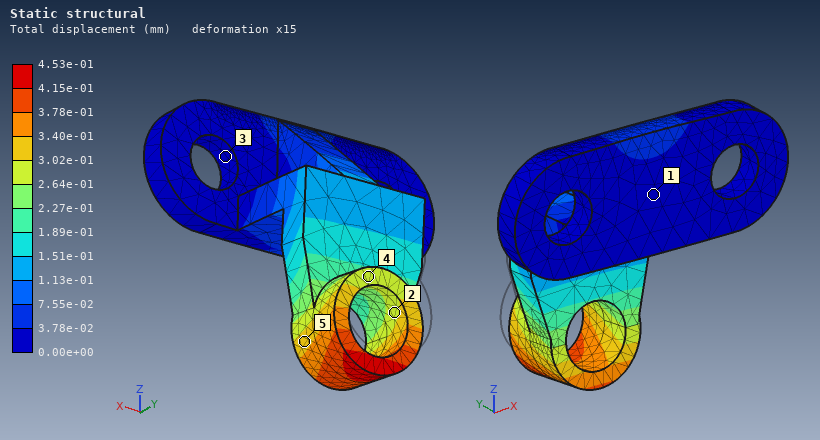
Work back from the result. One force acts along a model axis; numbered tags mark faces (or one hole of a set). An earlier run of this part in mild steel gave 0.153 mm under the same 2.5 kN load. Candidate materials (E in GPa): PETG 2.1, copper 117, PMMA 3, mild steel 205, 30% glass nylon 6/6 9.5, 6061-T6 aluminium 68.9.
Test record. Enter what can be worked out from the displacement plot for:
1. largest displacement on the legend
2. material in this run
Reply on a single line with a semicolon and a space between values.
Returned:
4.53e-01 mm; 6061-T6 aluminium
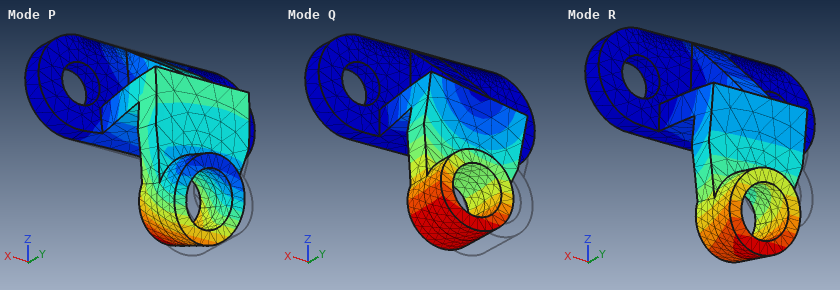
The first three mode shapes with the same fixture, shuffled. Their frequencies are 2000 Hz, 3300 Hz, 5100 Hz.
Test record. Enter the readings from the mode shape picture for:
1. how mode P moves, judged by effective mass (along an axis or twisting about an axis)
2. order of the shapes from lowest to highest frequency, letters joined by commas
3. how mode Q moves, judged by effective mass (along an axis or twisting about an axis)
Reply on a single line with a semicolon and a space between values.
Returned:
along Z; R, Q, P; along X
